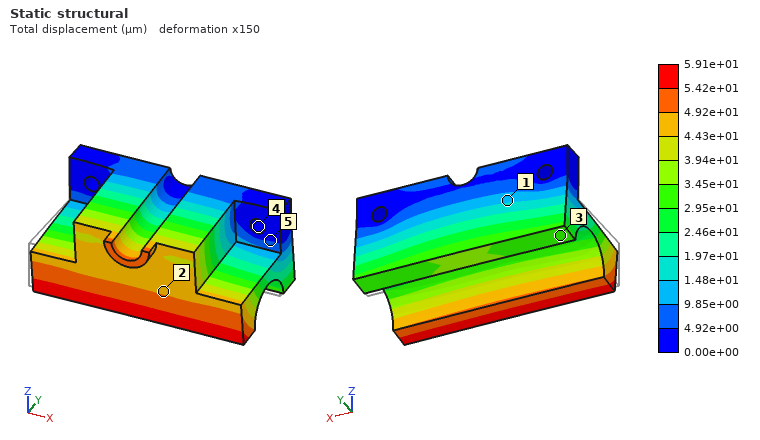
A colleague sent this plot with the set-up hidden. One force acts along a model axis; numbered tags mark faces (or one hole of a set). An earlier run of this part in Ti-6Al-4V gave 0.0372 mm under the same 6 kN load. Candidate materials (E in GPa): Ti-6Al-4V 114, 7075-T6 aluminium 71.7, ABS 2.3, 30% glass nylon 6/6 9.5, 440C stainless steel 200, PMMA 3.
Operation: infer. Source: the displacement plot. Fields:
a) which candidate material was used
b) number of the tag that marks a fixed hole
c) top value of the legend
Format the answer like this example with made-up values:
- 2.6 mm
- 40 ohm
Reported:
- 7075-T6 aluminium
- 4
- 5.91e+01 µm
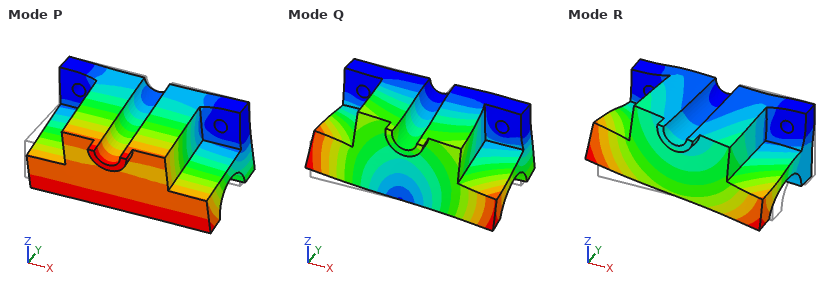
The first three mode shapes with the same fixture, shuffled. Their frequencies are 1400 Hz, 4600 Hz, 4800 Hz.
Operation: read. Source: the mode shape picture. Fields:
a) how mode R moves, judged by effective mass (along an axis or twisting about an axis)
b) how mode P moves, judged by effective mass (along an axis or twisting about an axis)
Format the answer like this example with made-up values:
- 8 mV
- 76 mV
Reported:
- along X
- along Z
